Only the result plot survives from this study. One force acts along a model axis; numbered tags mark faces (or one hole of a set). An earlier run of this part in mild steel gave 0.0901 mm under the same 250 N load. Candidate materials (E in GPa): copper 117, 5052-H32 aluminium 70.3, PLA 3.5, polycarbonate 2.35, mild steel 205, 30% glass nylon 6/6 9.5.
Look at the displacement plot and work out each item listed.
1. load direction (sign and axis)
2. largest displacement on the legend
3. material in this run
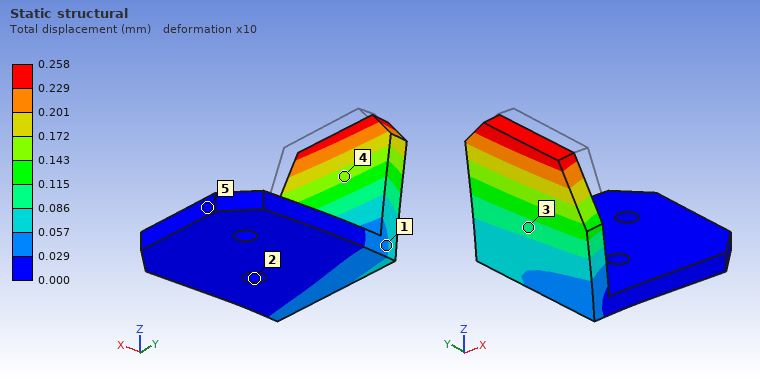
-X
0.258 mm
5052-H32 aluminium
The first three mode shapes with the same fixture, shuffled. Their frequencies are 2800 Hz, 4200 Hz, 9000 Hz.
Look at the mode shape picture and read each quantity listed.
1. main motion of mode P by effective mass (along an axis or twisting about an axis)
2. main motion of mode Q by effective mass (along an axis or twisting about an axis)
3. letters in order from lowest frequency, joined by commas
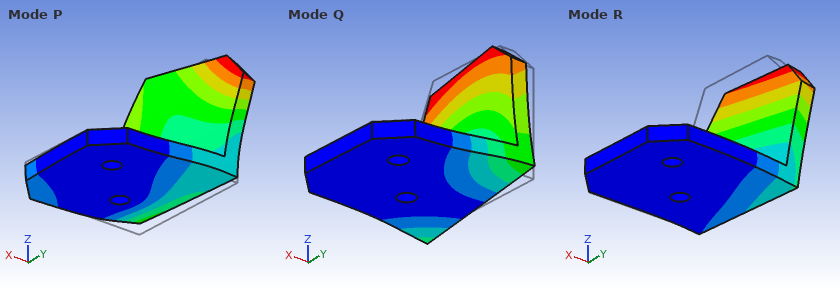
along Z
along Y
R, Q, P
